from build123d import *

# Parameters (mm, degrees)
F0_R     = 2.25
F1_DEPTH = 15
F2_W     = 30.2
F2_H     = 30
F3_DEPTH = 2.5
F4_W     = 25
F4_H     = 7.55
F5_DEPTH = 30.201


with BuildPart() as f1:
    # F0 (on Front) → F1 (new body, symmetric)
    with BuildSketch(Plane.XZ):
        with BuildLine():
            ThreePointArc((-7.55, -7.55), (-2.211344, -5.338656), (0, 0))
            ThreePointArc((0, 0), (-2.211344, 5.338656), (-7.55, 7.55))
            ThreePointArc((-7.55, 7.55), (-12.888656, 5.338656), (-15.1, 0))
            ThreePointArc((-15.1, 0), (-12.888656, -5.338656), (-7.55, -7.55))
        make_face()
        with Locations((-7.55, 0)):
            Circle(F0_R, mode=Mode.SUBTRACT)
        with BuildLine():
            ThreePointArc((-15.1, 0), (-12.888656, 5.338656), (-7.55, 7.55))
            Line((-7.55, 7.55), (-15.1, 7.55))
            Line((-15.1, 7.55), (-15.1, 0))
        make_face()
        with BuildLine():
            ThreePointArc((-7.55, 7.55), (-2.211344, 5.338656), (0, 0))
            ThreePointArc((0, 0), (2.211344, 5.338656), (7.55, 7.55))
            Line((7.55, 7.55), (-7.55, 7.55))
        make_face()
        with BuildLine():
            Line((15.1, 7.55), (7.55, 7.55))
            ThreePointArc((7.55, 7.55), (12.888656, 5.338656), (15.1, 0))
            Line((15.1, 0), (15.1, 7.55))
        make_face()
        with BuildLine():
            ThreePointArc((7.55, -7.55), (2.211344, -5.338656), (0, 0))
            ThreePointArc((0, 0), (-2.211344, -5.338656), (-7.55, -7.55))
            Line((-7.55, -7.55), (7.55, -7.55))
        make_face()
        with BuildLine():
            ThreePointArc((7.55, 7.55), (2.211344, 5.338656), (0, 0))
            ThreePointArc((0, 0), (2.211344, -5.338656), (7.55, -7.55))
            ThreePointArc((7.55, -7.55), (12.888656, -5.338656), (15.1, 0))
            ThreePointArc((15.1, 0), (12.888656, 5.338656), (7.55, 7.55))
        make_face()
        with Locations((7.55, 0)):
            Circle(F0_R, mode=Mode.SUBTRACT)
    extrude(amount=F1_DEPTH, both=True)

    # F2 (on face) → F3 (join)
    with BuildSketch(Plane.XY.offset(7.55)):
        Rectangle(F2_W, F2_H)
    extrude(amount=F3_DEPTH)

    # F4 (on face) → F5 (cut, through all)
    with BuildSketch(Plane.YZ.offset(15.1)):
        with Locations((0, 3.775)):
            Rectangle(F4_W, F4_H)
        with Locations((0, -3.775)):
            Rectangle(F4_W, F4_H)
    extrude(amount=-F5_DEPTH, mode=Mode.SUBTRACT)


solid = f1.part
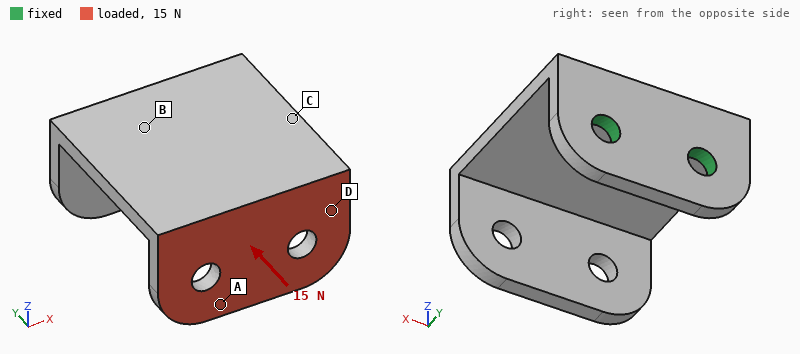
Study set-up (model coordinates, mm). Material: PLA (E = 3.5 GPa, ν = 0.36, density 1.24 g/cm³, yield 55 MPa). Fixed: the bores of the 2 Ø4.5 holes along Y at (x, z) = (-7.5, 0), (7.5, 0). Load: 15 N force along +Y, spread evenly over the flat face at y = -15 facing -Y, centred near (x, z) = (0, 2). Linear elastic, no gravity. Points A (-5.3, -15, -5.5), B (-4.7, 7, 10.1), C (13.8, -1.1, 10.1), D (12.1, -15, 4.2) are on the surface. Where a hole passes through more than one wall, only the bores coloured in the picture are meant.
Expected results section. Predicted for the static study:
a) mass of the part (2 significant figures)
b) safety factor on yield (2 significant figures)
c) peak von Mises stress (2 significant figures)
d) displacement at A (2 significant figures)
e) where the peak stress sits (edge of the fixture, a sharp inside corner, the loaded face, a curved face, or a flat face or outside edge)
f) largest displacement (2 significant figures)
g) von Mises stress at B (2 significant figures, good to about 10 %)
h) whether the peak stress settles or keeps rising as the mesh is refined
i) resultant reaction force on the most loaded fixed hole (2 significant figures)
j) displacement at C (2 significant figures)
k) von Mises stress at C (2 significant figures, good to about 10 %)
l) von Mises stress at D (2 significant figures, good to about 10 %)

5.3 g
15
3.6 MPa
0.49 mm
a flat face or outside edge
0.52 mm
2.8 MPa
settles
7.6 N
0.10 mm
3.3 MPa
1.6 MPa
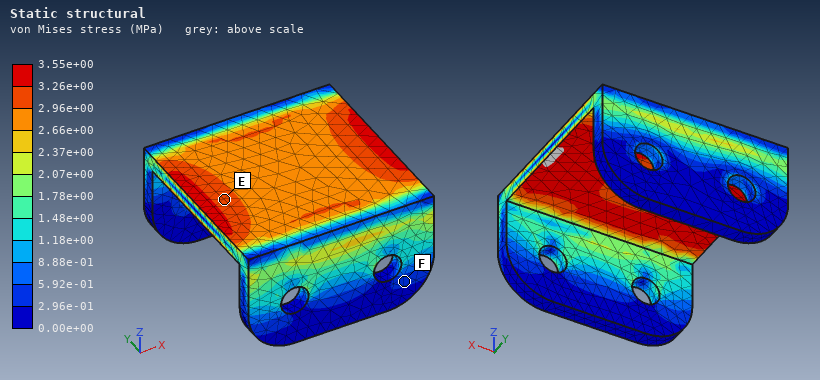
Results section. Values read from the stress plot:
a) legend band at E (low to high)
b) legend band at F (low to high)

2.96e+00 to 3.26e+00 MPa
2.96e-01 to 5.92e-01 MPa
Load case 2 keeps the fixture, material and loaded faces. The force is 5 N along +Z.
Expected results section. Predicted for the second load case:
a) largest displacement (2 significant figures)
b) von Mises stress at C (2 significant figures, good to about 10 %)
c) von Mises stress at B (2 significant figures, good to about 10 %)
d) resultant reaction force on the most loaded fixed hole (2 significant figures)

0.55 mm
2.3 MPa
3.1 MPa
2.8 N
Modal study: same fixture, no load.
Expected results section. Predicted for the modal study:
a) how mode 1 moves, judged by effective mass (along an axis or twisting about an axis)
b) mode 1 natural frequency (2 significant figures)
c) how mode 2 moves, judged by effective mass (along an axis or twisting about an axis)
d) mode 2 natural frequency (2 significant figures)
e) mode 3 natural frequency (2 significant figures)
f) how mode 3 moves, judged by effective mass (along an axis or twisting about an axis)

along Z
370 Hz
along X
780 Hz
1400 Hz
along Y
